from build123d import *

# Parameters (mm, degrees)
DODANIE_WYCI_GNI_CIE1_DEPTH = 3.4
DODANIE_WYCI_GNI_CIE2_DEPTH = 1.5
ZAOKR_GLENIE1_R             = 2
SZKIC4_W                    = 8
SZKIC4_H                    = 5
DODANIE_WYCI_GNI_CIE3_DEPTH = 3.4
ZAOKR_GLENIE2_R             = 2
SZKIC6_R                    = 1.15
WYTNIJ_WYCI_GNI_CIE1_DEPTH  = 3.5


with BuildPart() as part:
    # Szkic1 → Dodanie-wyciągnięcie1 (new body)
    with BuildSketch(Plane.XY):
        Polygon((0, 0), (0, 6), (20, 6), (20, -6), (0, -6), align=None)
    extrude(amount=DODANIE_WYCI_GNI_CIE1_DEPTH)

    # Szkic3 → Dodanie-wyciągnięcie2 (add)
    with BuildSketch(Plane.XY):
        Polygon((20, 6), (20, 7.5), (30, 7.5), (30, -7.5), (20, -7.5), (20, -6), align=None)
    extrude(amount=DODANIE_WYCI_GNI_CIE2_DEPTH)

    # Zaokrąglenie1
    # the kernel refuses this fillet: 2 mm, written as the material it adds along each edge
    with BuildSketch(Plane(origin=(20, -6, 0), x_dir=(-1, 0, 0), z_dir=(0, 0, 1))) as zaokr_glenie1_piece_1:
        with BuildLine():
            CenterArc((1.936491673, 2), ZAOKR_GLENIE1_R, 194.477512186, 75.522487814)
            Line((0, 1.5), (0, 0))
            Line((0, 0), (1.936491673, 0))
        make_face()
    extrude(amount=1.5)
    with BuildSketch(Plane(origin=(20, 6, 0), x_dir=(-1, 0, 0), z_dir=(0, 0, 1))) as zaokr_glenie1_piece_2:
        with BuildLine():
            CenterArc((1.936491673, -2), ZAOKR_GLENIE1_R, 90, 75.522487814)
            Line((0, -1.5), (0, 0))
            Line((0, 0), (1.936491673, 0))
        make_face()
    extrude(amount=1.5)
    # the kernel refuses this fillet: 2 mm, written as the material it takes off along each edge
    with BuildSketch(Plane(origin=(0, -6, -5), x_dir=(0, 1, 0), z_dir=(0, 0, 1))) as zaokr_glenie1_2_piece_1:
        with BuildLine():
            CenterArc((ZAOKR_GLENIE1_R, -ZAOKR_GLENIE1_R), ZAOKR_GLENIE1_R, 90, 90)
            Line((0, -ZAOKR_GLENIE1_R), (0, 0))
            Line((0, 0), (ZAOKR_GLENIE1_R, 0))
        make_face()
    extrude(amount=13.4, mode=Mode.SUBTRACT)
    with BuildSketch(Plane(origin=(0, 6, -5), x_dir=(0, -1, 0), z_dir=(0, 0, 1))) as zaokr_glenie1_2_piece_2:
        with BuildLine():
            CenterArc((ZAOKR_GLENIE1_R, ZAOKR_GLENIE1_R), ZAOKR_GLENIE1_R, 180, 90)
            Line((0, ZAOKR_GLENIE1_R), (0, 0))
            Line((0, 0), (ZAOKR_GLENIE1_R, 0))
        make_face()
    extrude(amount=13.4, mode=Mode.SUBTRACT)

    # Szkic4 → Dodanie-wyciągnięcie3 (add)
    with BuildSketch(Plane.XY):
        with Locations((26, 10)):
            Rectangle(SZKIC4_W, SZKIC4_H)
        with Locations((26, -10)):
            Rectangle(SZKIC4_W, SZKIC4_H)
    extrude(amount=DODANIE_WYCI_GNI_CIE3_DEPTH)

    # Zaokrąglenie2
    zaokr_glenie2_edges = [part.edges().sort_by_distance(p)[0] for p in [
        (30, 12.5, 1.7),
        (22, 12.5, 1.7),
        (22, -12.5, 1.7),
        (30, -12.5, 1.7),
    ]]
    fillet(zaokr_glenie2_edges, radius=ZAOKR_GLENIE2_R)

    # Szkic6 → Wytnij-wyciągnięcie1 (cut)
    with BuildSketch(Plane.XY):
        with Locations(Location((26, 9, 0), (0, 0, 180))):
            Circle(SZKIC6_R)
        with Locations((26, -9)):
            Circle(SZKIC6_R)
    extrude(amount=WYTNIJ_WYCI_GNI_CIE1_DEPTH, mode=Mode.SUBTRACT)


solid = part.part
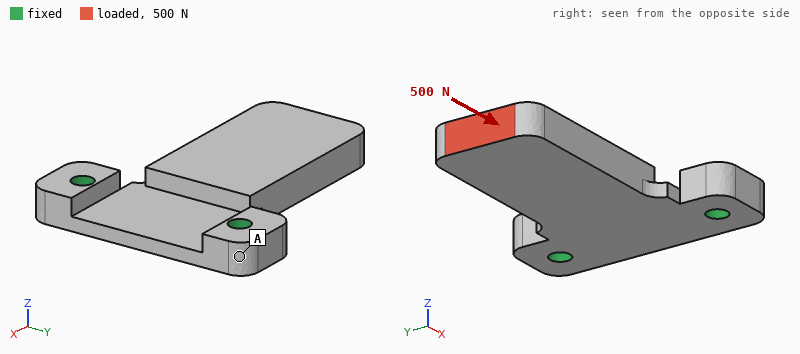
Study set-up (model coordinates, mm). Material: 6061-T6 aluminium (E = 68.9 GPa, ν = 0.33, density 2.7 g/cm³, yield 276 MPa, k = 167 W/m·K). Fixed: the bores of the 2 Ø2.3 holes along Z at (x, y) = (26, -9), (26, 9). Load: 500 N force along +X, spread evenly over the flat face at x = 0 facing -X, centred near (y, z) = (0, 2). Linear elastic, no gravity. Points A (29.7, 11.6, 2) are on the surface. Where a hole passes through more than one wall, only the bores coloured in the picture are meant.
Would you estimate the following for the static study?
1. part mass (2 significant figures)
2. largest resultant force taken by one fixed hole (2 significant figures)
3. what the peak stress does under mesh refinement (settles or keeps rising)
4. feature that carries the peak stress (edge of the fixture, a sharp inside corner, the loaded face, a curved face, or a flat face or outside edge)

3.4 g
270 N
keeps rising
a sharp inside corner
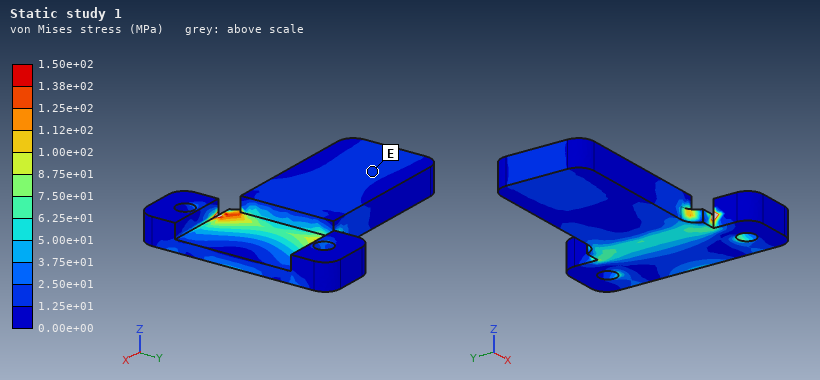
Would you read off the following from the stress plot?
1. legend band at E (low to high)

1.25e+01 to 2.50e+01 MPa
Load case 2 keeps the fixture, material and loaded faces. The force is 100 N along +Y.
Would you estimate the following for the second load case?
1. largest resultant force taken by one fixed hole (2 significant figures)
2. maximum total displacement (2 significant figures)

160 N
25 µm
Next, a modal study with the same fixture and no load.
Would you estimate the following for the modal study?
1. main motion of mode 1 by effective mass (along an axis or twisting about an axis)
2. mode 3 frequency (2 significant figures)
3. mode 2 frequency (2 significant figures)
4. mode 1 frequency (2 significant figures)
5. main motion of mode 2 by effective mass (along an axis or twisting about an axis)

along Z
13 kHz
12 kHz
1800 Hz
along Y
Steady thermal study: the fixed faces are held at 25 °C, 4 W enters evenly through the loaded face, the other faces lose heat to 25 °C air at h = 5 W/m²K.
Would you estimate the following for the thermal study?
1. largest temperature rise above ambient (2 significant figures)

21 K
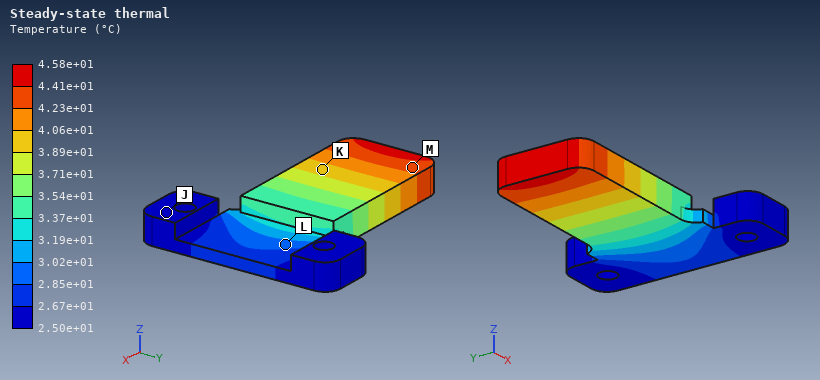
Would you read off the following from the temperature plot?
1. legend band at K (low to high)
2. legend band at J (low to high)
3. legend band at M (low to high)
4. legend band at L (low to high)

3.89e+01 to 4.06e+01 °C
2.50e+01 to 2.67e+01 °C
4.23e+01 to 4.41e+01 °C
2.85e+01 to 3.02e+01 °C
